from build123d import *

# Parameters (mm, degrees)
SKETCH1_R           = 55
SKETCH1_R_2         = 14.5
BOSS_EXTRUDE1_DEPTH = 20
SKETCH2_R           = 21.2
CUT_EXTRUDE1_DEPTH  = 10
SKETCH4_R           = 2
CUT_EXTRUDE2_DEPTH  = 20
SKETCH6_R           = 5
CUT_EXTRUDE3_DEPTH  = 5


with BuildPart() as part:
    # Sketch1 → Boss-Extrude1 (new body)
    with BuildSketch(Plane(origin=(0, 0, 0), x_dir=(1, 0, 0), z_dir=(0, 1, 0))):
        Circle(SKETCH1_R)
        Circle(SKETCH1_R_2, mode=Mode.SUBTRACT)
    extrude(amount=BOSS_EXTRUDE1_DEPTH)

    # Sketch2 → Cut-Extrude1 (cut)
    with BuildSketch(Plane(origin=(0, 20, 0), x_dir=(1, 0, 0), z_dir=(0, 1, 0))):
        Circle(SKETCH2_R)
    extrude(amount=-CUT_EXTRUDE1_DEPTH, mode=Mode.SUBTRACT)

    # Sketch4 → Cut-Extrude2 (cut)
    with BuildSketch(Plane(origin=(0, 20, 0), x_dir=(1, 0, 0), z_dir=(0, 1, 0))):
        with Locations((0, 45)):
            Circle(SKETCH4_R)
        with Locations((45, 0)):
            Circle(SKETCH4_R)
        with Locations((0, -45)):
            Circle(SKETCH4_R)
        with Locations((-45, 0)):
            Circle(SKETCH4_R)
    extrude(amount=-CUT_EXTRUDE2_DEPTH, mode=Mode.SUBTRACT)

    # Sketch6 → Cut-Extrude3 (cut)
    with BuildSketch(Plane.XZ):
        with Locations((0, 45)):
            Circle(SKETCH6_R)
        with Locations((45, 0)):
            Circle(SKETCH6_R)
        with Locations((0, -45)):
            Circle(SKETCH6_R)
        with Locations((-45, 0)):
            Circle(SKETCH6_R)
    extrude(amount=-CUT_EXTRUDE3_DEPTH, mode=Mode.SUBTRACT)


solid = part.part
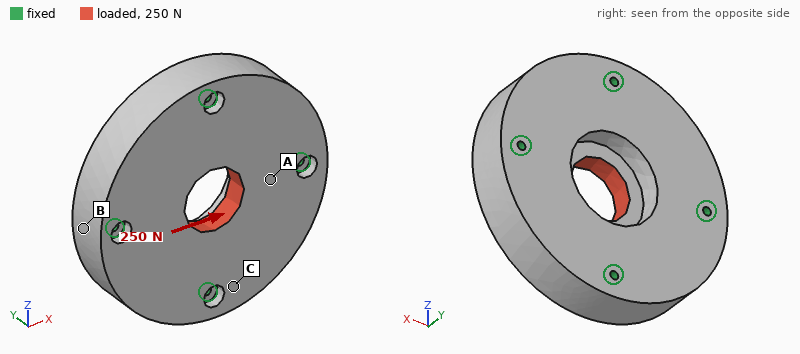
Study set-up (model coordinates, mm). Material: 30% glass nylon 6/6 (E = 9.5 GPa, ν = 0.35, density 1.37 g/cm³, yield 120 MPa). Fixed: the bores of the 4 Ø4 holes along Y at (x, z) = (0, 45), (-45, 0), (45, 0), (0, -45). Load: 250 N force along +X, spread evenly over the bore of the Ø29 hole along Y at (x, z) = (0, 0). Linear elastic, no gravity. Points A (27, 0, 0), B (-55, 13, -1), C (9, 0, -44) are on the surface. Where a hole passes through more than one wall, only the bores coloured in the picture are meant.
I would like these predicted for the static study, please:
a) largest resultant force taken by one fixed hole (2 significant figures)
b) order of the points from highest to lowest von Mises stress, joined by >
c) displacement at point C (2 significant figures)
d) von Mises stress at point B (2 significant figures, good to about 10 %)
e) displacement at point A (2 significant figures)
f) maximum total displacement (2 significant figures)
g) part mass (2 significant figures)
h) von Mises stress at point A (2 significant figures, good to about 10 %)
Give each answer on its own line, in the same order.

76 N
A > B > C
0.33 µm
0.15 MPa
0.74 µm
1.2 µm
230 g
0.30 MPa
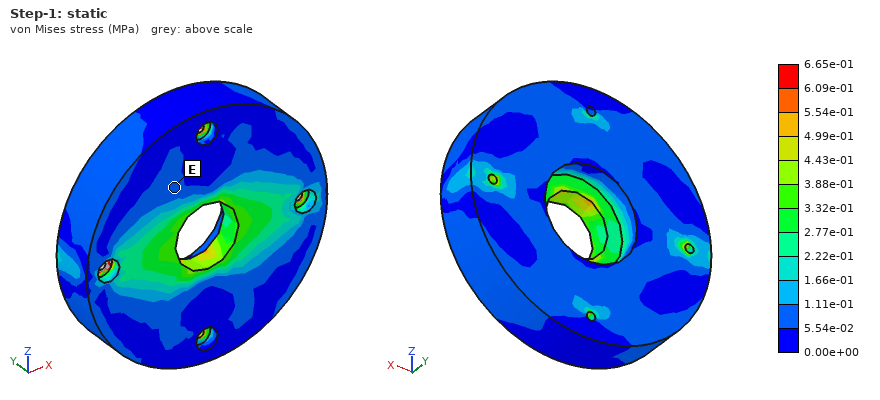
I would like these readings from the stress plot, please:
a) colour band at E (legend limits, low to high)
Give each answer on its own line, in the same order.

5.54e-02 to 1.11e-01 MPa
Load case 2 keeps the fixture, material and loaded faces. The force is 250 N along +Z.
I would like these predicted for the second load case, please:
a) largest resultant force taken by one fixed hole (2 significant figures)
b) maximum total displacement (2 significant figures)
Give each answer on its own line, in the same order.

76 N
1.2 µm
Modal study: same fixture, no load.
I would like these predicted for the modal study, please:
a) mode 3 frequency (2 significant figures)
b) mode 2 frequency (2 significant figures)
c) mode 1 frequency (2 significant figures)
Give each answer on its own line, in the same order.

5800 Hz
5800 Hz
5100 Hz
